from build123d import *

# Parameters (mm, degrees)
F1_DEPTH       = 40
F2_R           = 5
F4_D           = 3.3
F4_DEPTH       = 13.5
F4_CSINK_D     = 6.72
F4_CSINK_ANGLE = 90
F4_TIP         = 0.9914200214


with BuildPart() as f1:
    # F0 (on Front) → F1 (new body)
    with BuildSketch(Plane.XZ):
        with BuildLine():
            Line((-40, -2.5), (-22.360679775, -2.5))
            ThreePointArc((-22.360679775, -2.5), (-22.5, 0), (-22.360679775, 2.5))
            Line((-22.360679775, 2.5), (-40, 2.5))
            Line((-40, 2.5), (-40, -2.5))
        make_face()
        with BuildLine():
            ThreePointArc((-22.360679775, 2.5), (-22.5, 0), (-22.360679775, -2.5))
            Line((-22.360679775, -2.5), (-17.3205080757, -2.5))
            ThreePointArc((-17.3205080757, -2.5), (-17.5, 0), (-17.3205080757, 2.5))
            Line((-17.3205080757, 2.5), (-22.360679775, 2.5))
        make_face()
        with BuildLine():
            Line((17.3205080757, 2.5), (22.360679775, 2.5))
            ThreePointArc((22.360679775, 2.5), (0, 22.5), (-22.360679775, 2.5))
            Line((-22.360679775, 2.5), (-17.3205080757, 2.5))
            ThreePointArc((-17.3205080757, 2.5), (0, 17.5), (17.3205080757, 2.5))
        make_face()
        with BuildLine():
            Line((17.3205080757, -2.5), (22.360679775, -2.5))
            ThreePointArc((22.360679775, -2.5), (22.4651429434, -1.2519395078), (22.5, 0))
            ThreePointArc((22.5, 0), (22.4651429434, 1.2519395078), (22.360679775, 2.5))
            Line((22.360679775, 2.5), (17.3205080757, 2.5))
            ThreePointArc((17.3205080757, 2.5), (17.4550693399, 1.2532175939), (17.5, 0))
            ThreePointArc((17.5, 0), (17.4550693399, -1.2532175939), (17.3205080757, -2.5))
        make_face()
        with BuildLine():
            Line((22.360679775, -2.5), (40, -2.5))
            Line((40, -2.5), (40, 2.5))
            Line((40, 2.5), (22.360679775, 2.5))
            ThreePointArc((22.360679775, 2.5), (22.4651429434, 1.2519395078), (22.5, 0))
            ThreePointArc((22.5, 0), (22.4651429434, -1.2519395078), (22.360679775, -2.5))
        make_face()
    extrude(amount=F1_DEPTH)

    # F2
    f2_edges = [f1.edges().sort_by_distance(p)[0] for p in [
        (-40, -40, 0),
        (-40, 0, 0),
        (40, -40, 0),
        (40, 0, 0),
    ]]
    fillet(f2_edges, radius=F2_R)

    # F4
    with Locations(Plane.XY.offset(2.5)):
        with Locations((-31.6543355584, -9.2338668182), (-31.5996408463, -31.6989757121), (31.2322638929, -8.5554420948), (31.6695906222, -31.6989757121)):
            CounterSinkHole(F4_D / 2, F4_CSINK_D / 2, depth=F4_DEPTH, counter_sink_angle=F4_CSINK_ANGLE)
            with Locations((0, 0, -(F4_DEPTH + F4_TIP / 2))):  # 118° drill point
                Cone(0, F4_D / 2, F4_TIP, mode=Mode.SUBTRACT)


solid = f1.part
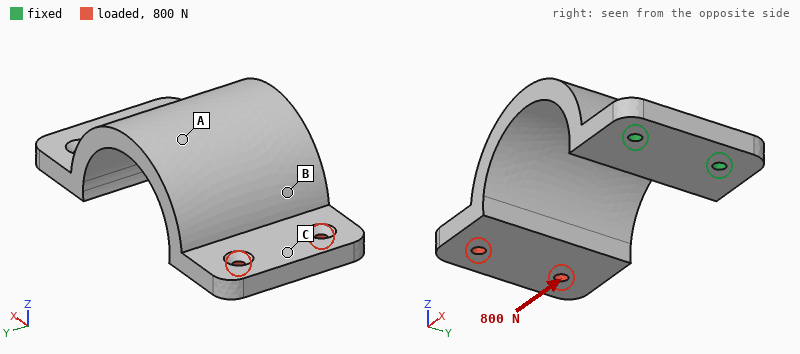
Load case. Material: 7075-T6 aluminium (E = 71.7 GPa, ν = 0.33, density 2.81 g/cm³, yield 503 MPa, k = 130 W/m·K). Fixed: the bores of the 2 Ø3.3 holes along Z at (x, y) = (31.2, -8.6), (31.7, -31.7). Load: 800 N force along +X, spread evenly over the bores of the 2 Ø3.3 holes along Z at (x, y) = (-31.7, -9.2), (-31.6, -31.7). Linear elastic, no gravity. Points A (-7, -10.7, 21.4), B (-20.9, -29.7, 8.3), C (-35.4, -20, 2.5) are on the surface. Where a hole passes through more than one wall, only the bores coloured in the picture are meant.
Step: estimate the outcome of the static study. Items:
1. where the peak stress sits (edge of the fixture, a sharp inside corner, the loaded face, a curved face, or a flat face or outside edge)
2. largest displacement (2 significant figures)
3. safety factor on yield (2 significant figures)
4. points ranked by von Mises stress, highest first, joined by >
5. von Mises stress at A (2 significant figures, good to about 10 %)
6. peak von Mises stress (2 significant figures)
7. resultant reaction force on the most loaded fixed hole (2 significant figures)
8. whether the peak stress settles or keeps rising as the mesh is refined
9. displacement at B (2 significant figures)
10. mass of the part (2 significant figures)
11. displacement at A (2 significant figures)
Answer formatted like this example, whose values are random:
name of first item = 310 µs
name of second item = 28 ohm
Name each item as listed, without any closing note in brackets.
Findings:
where the peak stress sits = a curved face
largest displacement = 0.96 mm
safety factor on yield = 4.7
points ranked by von Mises stress, highest first, joined by > = A > B > C
von Mises stress at A = 74 MPa
peak von Mises stress = 110 MPa
resultant reaction force on the most loaded fixed hole = 410 N
whether the peak stress settles or keeps rising as the mesh is refined = settles
displacement at B = 0.48 mm
mass of the part = 57 g
displacement at A = 0.22 mm
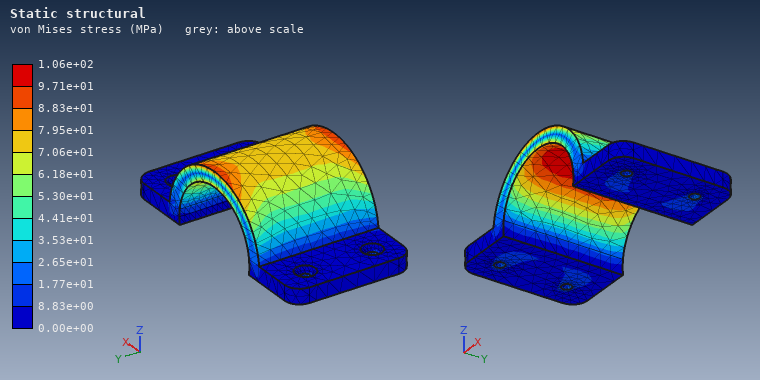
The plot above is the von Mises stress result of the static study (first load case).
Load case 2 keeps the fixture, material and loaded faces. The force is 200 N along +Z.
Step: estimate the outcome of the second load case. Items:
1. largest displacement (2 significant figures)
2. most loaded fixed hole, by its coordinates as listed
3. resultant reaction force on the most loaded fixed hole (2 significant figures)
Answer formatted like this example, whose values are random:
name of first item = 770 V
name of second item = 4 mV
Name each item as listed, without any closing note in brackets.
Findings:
largest displacement = 0.99 mm
most loaded fixed hole, by its coordinates as listed = (31.2, -8.6)
resultant reaction force on the most loaded fixed hole = 110 N
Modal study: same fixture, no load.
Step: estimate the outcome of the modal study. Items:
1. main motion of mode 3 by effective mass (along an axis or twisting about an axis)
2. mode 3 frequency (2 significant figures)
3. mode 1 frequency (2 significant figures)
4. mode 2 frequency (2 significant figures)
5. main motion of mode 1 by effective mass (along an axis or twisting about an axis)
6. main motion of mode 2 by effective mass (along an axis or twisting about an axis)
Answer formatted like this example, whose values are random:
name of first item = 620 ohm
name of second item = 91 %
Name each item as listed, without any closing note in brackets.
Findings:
main motion of mode 3 by effective mass = along X
mode 3 frequency = 1900 Hz
mode 1 frequency = 580 Hz
mode 2 frequency = 1200 Hz
main motion of mode 1 by effective mass = along Z
main motion of mode 2 by effective mass = along Y
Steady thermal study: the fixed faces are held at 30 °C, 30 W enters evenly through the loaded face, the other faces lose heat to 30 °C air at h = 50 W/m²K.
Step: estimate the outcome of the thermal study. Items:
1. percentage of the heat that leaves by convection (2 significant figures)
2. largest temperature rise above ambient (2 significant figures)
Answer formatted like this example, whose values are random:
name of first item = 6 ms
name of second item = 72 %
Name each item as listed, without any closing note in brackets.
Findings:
percentage of the heat that leaves by convection = 48 %
largest temperature rise above ambient = 69 K
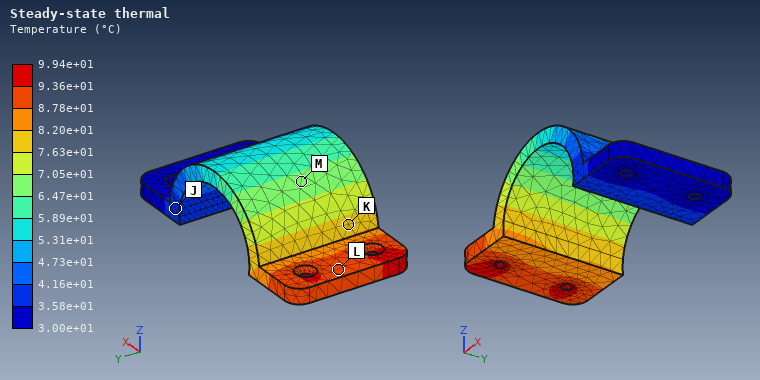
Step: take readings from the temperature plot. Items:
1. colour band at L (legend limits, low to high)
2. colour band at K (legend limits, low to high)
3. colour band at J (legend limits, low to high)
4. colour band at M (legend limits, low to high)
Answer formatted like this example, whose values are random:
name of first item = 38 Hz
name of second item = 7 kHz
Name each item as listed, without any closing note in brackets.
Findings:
colour band at L = 8.78e+01 to 9.36e+01 °C
colour band at K = 7.63e+01 to 8.20e+01 °C
colour band at J = 3.58e+01 to 4.16e+01 °C
colour band at M = 6.47e+01 to 7.05e+01 °C
